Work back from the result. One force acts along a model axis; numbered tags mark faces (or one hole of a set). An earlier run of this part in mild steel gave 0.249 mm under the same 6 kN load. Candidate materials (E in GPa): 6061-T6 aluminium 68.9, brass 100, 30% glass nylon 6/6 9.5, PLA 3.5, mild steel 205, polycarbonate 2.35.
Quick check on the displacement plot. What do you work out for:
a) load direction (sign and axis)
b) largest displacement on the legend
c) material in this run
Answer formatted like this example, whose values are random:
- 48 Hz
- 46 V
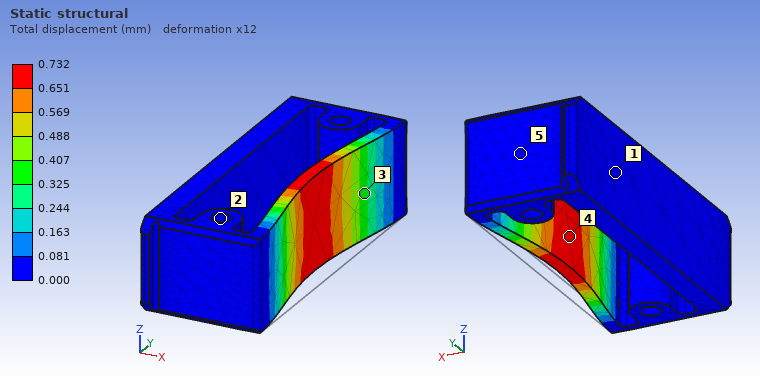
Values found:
- -X
- 0.732 mm
- 6061-T6 aluminium
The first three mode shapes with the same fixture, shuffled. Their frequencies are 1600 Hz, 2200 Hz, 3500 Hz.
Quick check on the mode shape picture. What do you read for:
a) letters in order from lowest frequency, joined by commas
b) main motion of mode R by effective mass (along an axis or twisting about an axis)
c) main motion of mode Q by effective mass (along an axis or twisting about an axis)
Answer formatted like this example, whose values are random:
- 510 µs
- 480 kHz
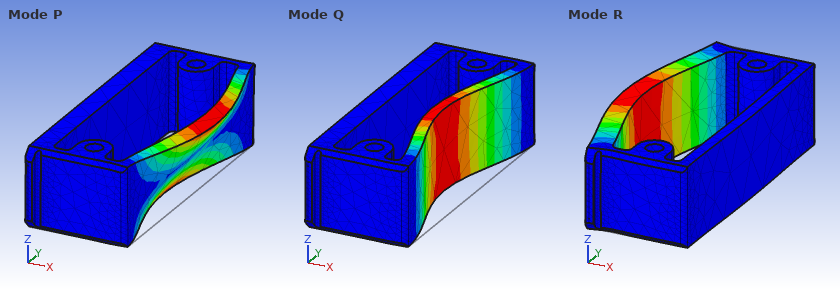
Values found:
- Q, R, P
- along X
- along X
